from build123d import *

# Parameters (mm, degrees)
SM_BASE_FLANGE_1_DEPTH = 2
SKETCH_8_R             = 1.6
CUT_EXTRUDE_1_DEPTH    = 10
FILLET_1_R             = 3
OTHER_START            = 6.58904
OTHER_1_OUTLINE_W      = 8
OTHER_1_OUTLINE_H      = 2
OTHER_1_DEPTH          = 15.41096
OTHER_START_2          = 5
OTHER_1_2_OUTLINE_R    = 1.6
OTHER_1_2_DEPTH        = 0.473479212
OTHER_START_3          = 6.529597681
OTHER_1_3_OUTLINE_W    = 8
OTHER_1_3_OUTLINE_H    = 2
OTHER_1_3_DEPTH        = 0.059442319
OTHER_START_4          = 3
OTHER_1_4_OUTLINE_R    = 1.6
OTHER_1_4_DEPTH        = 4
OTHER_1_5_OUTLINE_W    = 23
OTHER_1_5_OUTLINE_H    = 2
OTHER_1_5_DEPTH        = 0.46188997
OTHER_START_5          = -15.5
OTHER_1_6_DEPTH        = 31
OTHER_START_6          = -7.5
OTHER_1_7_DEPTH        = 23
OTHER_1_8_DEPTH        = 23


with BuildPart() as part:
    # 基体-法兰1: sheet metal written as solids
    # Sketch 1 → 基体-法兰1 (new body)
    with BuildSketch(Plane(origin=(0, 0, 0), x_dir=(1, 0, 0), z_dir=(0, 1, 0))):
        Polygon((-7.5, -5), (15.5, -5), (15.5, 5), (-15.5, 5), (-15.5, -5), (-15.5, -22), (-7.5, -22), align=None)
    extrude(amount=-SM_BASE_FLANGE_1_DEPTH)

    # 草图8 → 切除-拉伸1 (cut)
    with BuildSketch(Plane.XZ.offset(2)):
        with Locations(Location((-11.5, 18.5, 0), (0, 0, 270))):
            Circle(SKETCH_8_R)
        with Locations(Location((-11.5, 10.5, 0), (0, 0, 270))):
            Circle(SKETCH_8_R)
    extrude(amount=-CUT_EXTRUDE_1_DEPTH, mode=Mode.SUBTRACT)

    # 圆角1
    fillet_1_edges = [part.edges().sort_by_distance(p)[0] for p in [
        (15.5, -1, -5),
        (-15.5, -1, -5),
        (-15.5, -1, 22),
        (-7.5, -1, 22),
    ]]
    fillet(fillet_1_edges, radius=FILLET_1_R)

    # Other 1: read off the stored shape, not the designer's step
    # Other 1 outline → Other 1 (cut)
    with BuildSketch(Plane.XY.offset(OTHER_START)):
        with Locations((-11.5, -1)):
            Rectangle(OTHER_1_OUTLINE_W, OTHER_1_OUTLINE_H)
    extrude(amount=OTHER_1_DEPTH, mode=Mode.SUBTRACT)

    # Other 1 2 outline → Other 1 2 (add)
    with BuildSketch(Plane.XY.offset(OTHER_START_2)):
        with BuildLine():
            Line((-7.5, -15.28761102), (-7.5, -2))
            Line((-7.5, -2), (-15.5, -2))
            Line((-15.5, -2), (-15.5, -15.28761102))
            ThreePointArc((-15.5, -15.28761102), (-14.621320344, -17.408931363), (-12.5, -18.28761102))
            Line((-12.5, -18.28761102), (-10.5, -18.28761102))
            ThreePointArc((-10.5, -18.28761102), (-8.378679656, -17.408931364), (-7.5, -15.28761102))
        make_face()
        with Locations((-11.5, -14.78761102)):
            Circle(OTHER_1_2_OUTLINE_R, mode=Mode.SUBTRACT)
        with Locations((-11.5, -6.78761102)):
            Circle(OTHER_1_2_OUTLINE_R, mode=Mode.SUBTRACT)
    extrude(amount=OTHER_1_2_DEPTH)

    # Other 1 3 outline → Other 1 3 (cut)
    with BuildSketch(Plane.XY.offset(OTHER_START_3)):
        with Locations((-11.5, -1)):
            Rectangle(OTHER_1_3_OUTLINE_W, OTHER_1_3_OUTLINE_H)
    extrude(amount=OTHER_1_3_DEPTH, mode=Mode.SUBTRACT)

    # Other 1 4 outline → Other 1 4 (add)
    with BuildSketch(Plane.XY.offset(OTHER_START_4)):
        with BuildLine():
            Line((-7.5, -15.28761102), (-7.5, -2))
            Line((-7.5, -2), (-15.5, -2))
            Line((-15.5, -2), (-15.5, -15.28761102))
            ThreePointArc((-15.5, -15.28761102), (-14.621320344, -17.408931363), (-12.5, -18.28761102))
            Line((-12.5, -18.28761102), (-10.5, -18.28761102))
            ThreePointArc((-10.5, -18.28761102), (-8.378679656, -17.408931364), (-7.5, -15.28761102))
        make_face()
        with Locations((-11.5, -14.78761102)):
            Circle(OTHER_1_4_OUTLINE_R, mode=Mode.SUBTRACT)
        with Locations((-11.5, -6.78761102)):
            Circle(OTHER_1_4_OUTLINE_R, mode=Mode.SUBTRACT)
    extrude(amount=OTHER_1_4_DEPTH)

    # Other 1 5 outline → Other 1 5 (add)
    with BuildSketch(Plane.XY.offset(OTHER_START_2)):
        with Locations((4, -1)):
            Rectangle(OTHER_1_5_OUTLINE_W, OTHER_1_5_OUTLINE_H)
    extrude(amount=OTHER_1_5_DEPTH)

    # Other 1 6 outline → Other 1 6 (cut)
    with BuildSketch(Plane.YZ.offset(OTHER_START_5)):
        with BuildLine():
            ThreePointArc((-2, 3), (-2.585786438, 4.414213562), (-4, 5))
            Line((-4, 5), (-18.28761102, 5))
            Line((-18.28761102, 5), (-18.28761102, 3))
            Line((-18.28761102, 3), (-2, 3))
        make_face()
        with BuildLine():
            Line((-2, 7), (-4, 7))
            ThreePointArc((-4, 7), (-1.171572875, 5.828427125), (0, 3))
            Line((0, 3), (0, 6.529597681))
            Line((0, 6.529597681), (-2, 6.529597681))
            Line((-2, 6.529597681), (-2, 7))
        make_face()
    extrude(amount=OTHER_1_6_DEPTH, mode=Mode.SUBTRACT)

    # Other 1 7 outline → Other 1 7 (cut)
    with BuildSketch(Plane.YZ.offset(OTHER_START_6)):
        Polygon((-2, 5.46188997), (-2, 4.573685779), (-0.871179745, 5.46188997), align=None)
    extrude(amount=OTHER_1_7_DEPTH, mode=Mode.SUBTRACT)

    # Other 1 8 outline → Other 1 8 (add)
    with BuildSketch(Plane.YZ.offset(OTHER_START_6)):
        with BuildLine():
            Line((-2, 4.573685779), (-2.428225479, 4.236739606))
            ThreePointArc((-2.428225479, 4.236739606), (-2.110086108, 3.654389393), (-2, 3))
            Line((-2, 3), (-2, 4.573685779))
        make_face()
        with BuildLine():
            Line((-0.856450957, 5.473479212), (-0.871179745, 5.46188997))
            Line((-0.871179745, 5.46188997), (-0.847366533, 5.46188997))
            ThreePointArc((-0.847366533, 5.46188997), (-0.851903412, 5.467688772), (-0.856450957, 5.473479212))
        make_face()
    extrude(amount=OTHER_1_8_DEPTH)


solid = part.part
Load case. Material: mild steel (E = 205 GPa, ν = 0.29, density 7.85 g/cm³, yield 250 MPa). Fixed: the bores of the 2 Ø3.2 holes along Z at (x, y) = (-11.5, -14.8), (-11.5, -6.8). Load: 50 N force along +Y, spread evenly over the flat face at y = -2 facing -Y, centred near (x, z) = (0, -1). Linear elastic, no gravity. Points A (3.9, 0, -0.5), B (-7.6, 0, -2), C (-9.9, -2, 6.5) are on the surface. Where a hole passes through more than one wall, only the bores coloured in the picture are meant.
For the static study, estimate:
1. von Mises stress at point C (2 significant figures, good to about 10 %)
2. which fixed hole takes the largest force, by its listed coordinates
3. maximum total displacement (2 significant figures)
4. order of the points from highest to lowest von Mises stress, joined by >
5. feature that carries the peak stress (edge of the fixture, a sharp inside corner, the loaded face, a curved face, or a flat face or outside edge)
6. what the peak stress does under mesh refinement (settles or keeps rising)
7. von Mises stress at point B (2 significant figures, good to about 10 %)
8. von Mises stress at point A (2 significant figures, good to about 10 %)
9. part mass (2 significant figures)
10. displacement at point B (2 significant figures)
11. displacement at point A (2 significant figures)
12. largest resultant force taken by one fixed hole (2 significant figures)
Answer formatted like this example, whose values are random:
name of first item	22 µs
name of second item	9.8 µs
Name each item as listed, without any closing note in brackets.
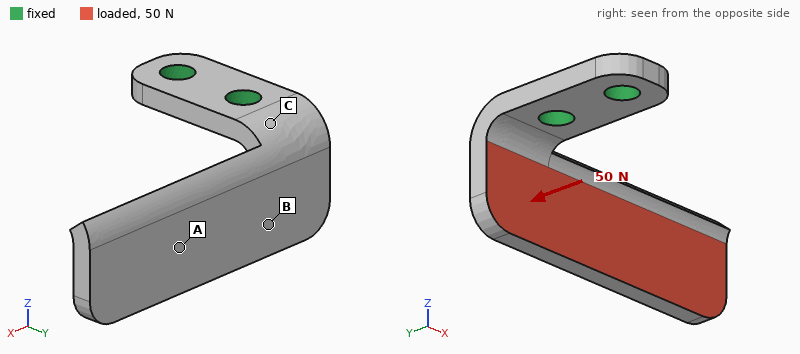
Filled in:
von Mises stress at point C	71 MPa
which fixed hole takes the largest force, by its listed coordinates	(-11.5, -6.8)
maximum total displacement	0.11 mm
order of the points from highest to lowest von Mises stress, joined by >	C > B > A
feature that carries the peak stress	a sharp inside corner
what the peak stress does under mesh refinement	keeps rising
von Mises stress at point B	48 MPa
von Mises stress at point A	17 MPa
part mass	6.6 g
displacement at point B	0.022 mm
displacement at point A	0.056 mm
largest resultant force taken by one fixed hole	52 N
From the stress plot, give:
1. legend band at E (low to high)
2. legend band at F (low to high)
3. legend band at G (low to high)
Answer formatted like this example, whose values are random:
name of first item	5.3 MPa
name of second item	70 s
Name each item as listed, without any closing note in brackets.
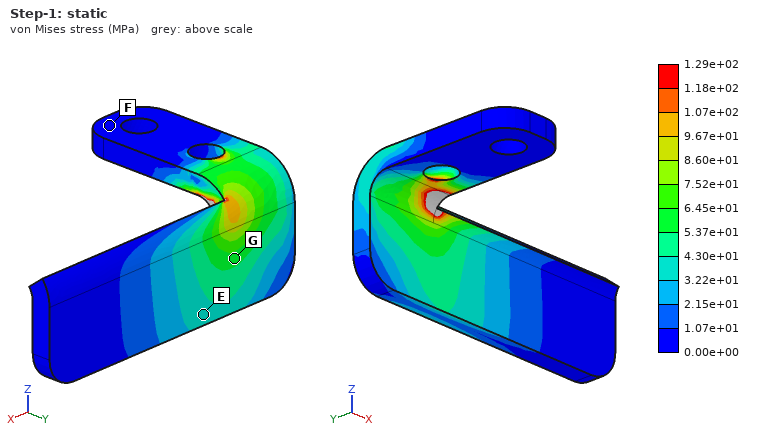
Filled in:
legend band at E	3.22e+01 to 4.30e+01 MPa
legend band at F	0.00e+00 to 1.07e+01 MPa
legend band at G	5.37e+01 to 6.45e+01 MPa
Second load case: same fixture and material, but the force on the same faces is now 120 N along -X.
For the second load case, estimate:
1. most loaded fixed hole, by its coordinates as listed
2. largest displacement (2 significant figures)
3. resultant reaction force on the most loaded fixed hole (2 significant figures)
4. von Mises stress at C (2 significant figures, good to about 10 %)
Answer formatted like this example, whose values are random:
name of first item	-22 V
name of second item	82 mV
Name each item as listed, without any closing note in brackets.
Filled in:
most loaded fixed hole, by its coordinates as listed	(-11.5, -6.8)
largest displacement	66 µm
resultant reaction force on the most loaded fixed hole	140 N
von Mises stress at C	69 MPa
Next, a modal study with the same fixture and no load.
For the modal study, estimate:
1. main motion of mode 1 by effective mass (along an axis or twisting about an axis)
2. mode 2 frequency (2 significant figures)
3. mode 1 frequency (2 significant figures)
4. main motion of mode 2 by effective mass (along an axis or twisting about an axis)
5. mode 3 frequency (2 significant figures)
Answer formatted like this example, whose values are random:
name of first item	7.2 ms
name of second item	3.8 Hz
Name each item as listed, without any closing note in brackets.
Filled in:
main motion of mode 1 by effective mass	along Y
mode 2 frequency	3000 Hz
mode 1 frequency	2000 Hz
main motion of mode 2 by effective mass	along Z
mode 3 frequency	6000 Hz
